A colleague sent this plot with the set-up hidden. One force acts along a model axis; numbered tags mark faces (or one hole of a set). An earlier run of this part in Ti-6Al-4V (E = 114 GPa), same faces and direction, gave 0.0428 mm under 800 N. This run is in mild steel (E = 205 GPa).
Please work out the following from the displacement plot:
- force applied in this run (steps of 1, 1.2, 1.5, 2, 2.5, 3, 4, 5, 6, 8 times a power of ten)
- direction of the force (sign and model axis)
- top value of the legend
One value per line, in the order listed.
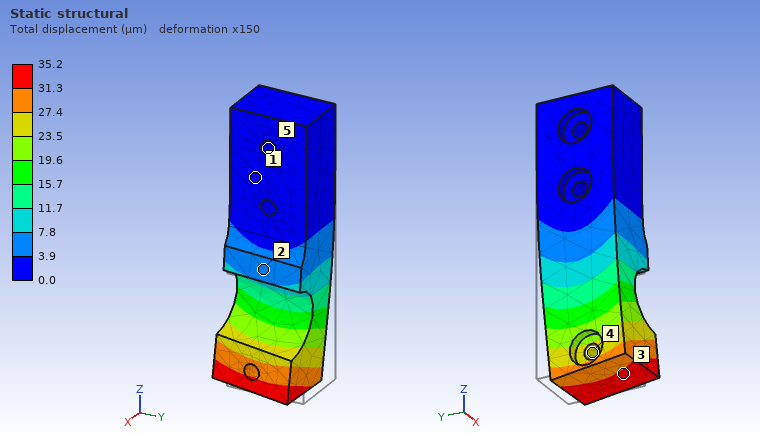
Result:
1.2 kN
-Y
35.2 µm
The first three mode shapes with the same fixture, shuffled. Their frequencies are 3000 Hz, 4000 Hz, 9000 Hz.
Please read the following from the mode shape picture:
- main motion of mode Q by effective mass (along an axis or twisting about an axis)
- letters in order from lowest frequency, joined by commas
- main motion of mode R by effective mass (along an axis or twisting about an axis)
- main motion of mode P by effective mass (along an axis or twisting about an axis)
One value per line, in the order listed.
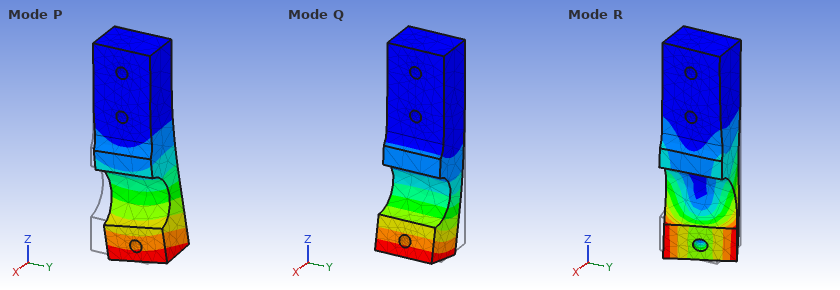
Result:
along X
Q, P, R
twisting about Z
along Y
